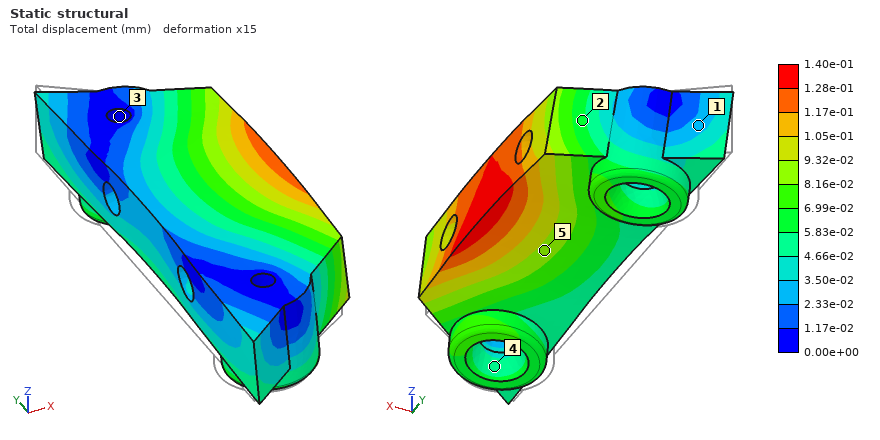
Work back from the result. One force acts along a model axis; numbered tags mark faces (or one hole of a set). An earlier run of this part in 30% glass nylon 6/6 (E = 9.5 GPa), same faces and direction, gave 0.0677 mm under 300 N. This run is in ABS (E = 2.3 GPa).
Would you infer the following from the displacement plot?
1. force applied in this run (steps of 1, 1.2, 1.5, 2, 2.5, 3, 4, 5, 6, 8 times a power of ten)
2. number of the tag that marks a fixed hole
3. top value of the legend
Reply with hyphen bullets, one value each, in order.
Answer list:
- 150 N
- 3
- 1.40e-01 mm
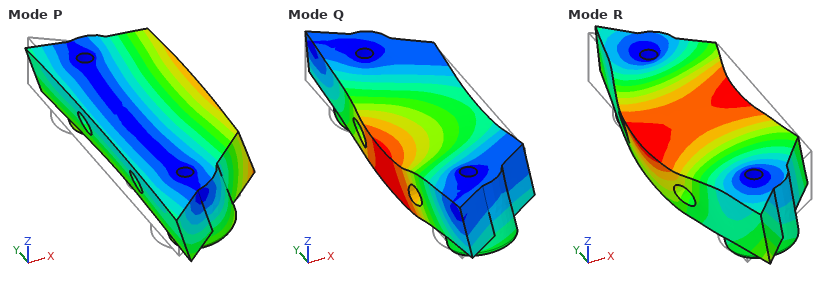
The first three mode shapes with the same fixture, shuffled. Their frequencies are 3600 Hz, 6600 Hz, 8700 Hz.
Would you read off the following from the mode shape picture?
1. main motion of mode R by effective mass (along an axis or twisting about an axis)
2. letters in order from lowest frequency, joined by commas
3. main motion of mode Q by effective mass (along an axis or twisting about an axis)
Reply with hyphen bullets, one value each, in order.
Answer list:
- along X
- P, Q, R
- along Z
